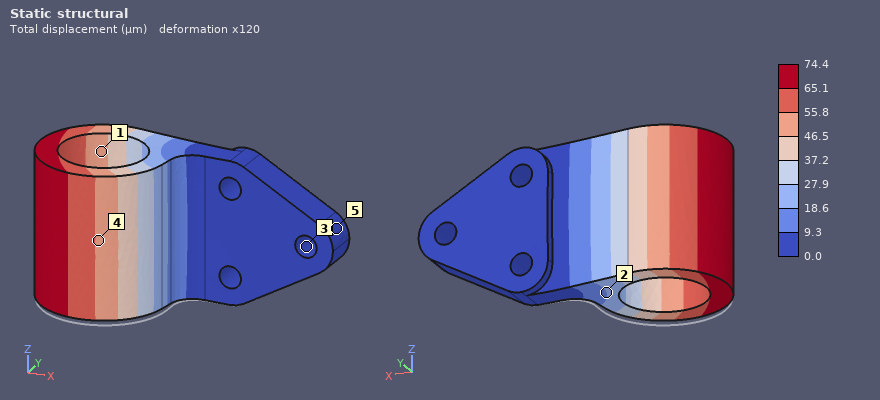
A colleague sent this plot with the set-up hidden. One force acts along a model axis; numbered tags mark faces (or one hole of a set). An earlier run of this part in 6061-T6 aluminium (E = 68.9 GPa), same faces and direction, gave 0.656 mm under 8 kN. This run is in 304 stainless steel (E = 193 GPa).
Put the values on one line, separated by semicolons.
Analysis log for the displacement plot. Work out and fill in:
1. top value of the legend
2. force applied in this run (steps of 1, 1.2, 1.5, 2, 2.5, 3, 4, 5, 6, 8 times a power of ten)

74.4 µm; 2.5 kN
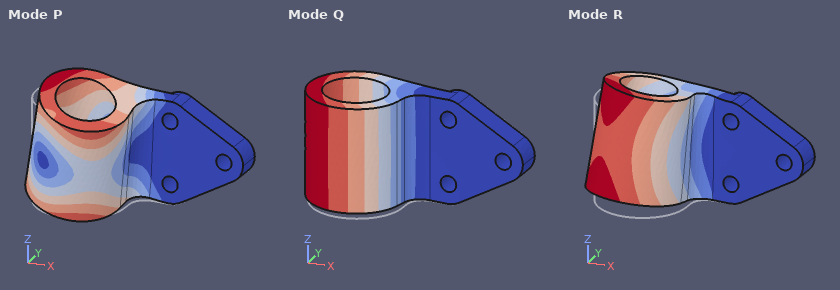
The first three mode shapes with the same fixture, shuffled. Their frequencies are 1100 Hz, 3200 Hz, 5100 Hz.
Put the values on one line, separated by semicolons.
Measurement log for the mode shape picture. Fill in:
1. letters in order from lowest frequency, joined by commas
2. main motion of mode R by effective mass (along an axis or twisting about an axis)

Q, R, P; along Z
